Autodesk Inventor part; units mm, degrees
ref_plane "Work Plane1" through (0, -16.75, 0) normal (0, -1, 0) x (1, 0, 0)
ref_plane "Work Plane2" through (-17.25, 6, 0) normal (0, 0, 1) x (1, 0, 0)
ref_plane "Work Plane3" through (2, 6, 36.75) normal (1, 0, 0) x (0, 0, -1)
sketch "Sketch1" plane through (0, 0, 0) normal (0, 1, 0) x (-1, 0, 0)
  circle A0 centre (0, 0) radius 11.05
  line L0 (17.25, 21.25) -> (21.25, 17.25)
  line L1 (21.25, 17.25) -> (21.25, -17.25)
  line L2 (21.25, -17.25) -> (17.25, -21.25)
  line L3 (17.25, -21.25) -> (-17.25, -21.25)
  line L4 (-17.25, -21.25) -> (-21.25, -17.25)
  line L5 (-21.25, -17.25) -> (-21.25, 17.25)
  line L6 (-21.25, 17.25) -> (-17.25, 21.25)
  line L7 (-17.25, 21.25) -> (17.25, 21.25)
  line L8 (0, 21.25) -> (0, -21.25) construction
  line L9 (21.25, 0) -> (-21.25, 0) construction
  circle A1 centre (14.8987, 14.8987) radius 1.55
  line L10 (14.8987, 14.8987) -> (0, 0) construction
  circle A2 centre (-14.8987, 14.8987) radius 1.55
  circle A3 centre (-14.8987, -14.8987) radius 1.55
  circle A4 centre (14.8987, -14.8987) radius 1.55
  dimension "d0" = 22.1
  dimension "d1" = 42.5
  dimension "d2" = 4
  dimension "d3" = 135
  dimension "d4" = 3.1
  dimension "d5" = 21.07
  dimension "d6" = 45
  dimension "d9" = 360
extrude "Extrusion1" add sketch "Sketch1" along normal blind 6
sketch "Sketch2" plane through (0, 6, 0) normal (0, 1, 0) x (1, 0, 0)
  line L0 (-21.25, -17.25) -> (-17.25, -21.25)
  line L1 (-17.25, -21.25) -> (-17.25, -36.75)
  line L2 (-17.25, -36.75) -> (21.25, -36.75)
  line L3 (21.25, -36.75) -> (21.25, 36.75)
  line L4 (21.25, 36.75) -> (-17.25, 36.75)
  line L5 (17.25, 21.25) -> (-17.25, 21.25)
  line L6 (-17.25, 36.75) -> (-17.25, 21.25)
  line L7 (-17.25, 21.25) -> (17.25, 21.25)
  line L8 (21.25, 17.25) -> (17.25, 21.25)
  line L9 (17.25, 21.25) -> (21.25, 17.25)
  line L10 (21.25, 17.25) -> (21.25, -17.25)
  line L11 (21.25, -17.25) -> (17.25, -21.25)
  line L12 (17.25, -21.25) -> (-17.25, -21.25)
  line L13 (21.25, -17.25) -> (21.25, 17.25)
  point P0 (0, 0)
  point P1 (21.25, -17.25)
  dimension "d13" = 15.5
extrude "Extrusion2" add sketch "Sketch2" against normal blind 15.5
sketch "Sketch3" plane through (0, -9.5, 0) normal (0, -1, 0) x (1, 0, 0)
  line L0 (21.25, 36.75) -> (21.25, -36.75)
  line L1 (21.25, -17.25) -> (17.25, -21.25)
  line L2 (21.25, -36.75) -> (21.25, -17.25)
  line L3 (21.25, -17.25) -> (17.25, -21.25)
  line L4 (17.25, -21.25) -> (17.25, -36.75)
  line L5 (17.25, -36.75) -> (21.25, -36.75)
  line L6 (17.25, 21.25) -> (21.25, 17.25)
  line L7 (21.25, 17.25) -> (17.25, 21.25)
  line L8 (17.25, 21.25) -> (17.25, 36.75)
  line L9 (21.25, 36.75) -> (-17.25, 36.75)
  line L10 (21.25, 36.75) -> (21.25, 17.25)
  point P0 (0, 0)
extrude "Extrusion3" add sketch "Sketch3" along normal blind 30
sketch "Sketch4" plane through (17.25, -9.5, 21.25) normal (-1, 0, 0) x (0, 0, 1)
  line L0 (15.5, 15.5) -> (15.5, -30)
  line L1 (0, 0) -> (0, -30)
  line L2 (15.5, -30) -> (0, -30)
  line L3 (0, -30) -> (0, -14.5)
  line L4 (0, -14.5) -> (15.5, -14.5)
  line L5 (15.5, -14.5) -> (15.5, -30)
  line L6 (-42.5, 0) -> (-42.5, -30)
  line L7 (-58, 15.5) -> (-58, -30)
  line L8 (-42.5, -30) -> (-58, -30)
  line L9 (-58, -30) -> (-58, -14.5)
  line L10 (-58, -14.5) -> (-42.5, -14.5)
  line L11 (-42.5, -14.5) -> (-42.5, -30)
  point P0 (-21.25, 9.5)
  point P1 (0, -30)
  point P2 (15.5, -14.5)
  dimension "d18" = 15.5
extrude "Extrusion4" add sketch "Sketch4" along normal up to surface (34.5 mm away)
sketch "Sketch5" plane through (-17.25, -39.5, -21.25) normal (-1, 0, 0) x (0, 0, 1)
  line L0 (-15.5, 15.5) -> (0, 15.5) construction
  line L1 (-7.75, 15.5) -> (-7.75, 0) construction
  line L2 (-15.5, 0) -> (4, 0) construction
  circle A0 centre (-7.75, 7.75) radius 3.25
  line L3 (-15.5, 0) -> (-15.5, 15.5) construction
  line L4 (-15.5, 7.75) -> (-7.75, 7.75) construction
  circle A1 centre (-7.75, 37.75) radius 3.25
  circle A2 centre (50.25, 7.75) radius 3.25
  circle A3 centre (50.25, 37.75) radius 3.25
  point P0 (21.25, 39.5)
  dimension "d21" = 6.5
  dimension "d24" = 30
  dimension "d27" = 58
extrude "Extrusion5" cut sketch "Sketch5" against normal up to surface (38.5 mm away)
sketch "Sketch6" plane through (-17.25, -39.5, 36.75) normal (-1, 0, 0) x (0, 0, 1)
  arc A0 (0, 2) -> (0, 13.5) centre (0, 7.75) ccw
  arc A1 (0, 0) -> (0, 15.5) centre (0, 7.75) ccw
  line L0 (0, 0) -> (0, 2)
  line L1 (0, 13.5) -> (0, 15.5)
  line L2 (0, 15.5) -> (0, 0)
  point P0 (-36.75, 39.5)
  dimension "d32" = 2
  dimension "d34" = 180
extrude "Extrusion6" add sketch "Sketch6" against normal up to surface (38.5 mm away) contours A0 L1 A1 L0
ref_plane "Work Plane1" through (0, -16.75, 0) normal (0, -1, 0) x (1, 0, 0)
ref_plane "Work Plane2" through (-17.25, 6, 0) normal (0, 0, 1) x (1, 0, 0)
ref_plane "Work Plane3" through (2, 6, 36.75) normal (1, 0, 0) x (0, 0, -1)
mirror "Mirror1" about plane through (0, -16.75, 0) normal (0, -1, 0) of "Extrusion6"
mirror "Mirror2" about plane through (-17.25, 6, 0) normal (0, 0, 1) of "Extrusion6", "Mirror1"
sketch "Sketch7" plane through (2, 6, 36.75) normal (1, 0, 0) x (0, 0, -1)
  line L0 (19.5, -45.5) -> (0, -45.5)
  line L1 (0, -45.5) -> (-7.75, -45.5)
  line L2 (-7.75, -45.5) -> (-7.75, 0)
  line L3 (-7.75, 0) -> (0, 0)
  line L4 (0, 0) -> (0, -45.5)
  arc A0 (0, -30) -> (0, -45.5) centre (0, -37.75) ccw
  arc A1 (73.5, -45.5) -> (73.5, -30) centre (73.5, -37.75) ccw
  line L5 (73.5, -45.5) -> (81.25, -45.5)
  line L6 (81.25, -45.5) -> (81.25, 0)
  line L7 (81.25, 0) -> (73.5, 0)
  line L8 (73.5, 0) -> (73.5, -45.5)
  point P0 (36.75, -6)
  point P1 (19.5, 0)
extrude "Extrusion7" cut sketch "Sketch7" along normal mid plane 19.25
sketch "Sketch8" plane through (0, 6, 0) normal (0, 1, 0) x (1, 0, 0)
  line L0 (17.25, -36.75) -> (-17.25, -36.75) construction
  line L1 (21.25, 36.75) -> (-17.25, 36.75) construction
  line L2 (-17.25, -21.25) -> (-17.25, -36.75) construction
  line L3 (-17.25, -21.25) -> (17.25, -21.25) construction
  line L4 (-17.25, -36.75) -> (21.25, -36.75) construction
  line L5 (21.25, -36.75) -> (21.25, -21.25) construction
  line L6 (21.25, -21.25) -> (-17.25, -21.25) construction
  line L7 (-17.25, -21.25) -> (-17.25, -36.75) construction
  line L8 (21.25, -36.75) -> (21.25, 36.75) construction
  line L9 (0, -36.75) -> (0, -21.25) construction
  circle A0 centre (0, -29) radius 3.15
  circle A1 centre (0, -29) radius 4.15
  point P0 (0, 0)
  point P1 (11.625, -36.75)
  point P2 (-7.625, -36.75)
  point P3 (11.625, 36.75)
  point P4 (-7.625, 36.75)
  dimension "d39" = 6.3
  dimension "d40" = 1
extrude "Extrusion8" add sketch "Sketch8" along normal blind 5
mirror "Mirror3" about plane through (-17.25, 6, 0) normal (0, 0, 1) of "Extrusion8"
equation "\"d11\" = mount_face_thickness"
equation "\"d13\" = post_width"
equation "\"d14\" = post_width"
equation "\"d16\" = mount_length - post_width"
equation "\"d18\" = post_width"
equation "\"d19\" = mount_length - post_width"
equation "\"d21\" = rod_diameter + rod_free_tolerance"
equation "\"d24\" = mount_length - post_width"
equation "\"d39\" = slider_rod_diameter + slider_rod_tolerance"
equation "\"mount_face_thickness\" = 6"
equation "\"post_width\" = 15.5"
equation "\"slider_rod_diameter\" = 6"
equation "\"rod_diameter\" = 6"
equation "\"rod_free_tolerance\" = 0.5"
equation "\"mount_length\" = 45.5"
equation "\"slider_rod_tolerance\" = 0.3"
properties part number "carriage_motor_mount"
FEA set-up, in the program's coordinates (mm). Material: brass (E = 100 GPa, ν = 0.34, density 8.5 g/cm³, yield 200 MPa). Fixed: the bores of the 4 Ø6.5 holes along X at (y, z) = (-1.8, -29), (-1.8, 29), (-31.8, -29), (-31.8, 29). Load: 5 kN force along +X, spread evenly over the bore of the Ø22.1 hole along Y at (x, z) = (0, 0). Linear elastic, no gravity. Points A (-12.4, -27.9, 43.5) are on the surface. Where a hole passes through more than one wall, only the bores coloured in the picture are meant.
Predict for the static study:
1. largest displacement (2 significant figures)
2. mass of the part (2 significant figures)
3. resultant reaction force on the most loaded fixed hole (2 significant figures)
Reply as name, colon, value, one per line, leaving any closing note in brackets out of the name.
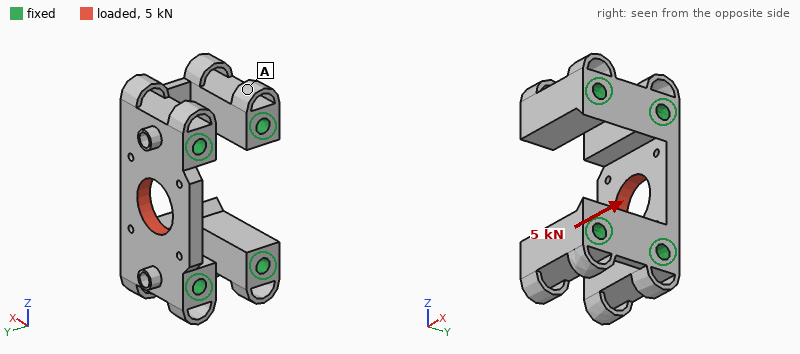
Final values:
largest displacement: 9.4 µm
mass of the part: 390 g
resultant reaction force on the most loaded fixed hole: 2.5 kN
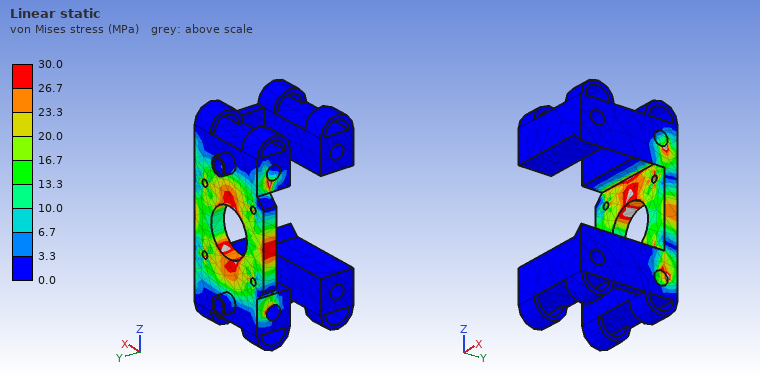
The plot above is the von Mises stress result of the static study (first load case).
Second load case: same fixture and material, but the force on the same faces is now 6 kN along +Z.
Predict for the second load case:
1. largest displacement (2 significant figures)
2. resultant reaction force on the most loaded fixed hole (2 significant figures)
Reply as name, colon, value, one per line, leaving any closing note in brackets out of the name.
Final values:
largest displacement: 4.8 µm
resultant reaction force on the most loaded fixed hole: 3.0 kN
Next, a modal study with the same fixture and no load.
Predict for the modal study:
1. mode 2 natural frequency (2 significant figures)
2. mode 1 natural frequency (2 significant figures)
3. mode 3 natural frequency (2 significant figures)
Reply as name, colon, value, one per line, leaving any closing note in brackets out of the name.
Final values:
mode 2 natural frequency: 10000 Hz
mode 1 natural frequency: 8400 Hz
mode 3 natural frequency: 18 kHz
